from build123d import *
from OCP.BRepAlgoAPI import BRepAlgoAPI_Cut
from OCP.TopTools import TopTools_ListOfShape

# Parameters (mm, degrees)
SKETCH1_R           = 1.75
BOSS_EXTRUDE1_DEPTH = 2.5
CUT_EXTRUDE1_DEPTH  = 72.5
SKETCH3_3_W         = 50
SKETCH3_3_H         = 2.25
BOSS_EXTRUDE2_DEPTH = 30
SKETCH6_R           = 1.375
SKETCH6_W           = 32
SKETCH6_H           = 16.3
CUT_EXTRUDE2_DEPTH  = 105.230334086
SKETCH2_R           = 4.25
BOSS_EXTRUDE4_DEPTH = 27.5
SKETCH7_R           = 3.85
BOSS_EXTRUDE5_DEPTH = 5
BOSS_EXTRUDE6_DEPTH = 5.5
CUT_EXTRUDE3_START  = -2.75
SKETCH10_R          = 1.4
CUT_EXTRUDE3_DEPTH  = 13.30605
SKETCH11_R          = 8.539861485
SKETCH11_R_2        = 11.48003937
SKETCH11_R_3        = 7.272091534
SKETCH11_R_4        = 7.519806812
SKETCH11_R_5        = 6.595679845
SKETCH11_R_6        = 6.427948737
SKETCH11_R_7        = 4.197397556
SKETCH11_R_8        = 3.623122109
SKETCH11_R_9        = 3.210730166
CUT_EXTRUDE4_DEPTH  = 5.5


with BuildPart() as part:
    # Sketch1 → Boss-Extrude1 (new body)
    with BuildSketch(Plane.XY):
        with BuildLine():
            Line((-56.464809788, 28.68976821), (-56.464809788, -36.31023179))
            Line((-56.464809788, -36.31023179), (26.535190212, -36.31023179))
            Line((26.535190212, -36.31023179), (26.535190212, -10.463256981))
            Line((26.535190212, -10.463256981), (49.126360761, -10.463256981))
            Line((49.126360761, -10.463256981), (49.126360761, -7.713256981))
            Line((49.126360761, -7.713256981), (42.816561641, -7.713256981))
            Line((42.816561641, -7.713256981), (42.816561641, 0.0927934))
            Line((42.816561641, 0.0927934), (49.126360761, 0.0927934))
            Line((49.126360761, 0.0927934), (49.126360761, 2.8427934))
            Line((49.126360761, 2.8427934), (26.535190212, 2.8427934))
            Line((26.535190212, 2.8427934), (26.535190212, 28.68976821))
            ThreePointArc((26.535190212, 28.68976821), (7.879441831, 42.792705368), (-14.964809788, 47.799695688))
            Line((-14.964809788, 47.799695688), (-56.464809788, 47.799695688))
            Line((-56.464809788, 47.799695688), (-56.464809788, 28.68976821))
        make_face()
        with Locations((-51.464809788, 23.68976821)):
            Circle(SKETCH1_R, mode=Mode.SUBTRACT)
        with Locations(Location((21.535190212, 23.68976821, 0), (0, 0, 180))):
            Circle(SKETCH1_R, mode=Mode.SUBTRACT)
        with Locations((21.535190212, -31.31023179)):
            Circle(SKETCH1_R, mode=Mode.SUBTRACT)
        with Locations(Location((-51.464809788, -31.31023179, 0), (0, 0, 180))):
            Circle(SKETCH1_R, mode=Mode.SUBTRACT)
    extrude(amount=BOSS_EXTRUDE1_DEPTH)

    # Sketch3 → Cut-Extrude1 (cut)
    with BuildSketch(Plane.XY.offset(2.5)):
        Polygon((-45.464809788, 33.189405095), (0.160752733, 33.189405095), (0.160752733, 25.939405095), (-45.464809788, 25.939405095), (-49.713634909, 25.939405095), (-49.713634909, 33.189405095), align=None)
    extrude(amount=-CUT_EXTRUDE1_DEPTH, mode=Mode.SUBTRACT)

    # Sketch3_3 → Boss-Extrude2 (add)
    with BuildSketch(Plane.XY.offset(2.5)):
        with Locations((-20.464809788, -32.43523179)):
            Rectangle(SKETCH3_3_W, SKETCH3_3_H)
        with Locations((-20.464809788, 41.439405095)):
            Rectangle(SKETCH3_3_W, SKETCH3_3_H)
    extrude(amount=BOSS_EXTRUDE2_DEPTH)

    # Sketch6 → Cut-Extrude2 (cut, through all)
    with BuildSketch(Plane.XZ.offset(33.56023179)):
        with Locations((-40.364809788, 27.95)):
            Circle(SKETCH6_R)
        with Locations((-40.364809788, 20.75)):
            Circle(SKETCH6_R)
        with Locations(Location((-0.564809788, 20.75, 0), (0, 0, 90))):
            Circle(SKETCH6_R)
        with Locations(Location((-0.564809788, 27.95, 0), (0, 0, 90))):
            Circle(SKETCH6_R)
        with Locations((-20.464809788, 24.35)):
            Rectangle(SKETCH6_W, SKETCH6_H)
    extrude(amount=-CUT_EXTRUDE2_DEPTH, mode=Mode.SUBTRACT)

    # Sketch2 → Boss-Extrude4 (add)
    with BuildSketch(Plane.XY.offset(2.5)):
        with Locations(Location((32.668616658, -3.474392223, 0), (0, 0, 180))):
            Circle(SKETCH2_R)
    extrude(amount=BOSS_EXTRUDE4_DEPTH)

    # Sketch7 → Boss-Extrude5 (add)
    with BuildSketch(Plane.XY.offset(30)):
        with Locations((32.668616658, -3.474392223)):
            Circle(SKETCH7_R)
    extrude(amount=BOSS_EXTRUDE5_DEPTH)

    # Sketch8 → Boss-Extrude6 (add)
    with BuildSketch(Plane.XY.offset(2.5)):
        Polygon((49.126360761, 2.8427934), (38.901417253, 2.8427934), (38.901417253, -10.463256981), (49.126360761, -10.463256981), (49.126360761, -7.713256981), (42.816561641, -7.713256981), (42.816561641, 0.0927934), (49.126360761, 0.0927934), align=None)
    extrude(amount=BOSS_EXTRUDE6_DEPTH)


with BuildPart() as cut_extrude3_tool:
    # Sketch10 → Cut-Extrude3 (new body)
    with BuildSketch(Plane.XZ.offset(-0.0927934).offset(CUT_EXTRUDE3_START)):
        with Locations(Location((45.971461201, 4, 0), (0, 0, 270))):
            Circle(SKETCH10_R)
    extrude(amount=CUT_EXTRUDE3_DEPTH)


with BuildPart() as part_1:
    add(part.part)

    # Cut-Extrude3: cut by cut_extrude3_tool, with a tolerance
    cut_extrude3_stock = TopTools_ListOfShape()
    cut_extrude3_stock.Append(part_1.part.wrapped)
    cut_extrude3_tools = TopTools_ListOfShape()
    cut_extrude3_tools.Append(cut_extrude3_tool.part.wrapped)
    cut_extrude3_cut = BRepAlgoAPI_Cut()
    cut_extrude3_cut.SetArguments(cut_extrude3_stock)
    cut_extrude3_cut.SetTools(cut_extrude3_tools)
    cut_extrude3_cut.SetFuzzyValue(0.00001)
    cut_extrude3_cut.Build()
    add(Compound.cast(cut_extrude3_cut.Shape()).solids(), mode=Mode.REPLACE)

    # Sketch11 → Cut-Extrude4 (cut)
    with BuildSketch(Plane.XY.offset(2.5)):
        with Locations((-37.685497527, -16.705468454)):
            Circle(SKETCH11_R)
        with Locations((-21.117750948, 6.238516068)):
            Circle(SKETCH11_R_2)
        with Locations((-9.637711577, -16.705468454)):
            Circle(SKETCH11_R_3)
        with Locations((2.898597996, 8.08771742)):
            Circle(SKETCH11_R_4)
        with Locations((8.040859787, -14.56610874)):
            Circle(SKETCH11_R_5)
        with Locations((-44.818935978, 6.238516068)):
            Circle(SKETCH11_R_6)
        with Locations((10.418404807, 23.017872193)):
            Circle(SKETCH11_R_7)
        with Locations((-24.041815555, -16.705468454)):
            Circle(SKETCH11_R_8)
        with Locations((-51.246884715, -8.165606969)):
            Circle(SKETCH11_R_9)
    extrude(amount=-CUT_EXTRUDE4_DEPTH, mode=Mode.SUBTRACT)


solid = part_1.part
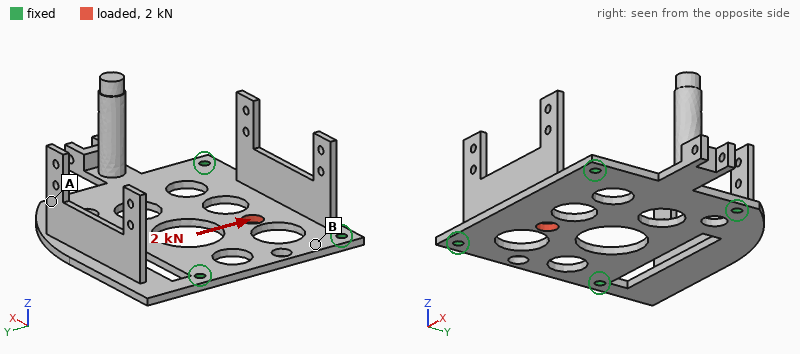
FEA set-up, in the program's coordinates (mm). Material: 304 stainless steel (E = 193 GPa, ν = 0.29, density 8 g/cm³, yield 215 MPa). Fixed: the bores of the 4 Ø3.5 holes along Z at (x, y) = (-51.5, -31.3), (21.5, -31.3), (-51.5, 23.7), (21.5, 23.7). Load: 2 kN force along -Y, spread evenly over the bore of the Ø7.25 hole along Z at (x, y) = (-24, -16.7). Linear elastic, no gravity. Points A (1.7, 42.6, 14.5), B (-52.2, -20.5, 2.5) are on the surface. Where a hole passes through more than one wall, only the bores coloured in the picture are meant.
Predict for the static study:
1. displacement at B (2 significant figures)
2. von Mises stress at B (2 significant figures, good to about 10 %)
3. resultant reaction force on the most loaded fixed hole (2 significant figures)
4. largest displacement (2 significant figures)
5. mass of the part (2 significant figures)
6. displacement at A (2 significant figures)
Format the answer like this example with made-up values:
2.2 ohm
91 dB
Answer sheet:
2.3 µm
21 MPa
670 N
15 µm
160 g
3.2 µm
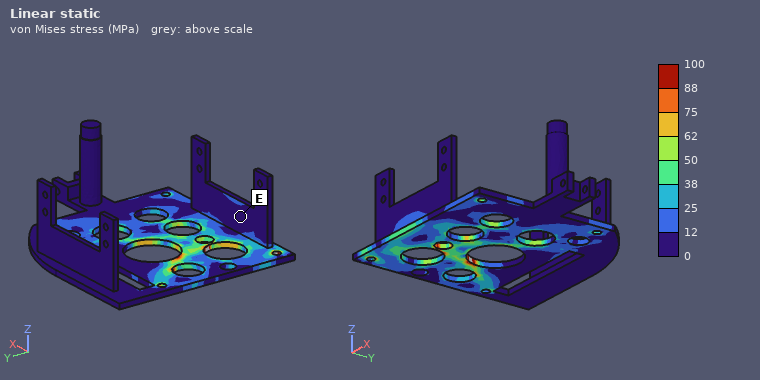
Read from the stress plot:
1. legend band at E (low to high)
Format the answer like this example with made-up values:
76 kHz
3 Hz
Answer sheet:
0 to 12 MPa
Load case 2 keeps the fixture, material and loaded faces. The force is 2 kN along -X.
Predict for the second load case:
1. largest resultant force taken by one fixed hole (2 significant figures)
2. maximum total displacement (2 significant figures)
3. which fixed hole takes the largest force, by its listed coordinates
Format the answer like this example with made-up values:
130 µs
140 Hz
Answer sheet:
820 N
11 µm
(-51.5, -31.3)
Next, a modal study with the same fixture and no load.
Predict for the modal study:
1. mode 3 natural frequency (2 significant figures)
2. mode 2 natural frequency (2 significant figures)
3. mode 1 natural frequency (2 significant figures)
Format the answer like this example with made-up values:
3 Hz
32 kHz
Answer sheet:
1600 Hz
1000 Hz
840 Hz
